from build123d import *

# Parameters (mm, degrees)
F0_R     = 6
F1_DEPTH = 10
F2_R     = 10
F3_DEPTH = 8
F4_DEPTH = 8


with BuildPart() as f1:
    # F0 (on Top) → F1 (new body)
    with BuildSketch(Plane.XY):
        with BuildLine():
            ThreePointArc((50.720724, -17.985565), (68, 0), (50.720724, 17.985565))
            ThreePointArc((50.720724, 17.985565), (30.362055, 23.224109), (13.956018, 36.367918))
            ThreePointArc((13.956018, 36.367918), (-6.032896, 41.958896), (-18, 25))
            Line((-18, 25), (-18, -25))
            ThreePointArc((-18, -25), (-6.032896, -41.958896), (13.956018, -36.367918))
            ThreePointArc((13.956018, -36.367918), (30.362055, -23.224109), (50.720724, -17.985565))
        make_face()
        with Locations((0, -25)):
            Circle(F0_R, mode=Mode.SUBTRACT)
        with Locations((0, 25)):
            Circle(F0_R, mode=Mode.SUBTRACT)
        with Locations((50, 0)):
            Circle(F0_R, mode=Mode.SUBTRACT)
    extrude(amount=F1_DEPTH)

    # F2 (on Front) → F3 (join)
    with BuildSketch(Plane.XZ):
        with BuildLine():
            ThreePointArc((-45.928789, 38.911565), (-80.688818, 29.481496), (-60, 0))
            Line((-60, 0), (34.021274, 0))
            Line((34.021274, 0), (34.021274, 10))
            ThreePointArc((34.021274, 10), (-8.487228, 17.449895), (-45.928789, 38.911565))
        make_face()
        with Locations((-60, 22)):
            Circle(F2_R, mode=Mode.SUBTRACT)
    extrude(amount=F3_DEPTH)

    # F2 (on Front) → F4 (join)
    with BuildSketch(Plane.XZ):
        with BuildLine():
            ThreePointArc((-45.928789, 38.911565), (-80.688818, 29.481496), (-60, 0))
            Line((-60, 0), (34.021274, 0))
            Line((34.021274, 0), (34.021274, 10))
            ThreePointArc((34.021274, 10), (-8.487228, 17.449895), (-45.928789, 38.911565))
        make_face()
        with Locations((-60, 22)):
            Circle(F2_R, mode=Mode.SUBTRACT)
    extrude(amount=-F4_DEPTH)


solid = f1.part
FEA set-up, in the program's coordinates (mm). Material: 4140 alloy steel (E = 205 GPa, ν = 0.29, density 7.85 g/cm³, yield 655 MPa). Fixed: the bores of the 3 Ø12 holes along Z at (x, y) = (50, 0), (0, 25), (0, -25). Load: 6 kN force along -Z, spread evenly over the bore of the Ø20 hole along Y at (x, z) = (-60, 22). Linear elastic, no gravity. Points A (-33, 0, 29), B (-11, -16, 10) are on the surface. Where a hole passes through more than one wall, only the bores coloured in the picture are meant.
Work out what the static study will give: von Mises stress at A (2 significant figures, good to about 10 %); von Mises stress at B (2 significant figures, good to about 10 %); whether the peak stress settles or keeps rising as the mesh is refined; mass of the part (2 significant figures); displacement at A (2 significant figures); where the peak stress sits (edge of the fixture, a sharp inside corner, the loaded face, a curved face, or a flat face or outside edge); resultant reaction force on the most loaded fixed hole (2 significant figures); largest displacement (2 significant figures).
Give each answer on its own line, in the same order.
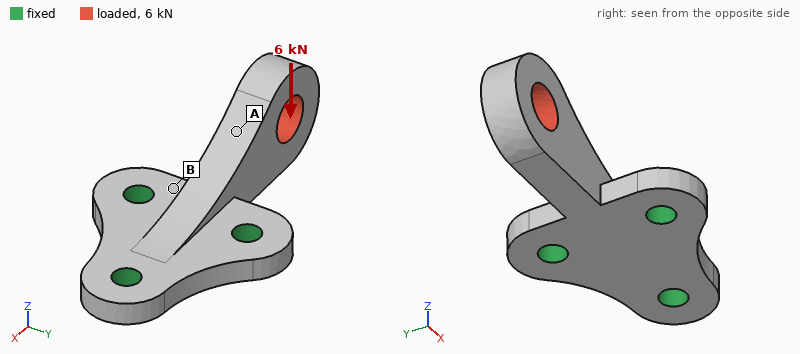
48 MPa
170 MPa
keeps rising
610 g
0.19 mm
edge of the fixture
5.6 kN
0.44 mm
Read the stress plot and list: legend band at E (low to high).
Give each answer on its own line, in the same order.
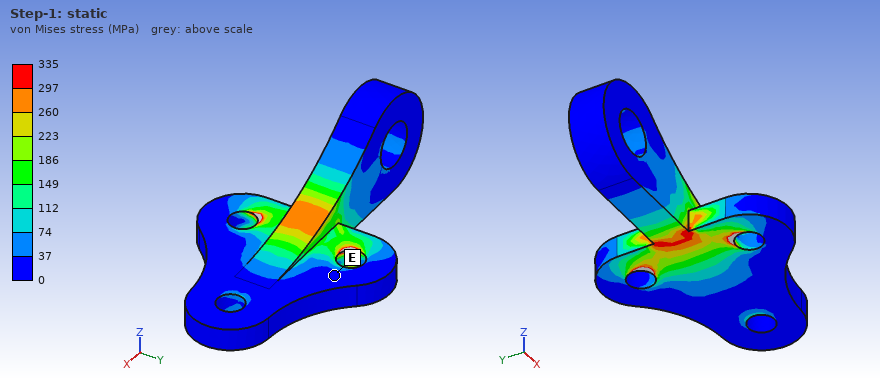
0 to 37 MPa
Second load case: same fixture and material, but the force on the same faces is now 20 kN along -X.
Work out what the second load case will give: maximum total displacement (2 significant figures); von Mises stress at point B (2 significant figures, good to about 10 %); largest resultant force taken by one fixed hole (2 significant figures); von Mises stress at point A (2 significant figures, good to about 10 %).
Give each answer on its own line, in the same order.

0.42 mm
210 MPa
7.0 kN
110 MPa
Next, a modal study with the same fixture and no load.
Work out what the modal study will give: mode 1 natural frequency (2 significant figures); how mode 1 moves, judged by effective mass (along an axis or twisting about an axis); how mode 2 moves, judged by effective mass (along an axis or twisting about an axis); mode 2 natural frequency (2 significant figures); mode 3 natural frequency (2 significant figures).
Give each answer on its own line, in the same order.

1600 Hz
along Z
along Y
2000 Hz
5400 Hz
